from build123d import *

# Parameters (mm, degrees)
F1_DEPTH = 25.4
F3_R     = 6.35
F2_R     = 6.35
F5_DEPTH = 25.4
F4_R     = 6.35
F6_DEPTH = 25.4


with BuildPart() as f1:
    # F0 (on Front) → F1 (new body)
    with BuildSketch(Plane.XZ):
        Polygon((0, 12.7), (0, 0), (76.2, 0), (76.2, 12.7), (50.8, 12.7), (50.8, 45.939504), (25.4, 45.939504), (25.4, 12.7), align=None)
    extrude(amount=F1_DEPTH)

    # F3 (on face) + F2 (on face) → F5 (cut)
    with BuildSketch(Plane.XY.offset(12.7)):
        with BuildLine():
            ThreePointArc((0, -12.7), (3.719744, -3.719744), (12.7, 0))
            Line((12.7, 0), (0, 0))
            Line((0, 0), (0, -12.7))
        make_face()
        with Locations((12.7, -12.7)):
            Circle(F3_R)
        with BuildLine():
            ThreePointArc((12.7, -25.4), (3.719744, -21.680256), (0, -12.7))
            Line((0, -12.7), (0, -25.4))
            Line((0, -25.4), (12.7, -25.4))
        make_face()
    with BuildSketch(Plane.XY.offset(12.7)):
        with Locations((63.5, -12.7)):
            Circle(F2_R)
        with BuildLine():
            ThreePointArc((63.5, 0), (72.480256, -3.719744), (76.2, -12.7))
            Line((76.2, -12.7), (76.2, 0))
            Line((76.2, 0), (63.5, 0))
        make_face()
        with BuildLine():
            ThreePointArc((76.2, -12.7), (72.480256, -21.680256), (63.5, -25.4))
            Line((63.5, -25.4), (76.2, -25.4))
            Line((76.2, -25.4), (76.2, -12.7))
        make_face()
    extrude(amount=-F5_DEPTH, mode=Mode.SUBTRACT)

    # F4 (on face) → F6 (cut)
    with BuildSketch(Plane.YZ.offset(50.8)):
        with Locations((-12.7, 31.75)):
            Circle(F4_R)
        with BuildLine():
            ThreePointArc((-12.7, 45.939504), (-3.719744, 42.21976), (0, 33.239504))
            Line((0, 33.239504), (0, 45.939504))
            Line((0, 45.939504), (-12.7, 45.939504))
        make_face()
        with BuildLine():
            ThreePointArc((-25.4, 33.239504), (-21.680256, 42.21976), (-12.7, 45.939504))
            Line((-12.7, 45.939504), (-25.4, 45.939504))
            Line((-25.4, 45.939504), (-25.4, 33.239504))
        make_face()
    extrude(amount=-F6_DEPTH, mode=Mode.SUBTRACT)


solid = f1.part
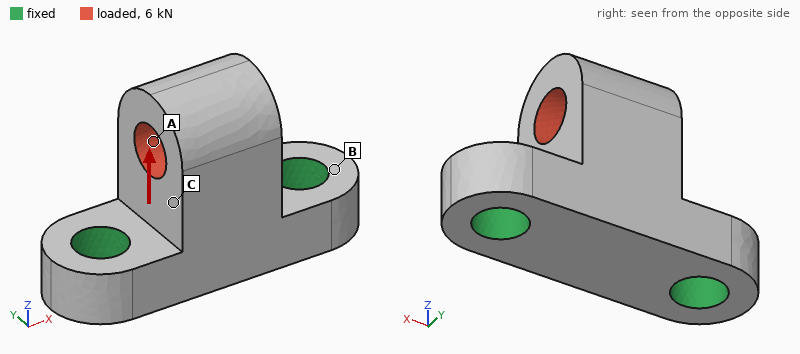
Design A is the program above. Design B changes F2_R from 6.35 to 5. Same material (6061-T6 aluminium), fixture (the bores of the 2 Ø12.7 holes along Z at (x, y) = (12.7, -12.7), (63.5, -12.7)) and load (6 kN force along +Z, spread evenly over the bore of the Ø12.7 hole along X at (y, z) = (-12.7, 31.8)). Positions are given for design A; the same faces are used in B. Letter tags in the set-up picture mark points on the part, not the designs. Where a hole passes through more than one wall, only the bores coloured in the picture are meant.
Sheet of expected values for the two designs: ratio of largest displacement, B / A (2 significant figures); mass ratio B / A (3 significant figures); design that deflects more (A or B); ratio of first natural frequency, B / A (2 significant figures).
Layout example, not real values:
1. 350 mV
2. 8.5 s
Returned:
1. 1.1
2. 1.02
3. B
4. 0.97
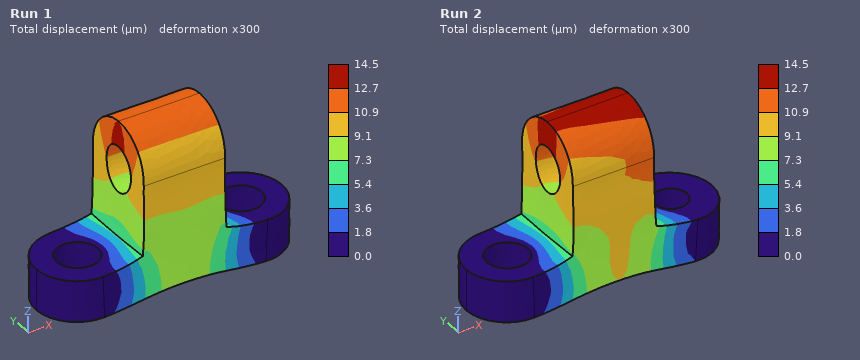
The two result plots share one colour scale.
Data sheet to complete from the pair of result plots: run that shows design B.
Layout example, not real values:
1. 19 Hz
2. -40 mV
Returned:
1. Run 2
